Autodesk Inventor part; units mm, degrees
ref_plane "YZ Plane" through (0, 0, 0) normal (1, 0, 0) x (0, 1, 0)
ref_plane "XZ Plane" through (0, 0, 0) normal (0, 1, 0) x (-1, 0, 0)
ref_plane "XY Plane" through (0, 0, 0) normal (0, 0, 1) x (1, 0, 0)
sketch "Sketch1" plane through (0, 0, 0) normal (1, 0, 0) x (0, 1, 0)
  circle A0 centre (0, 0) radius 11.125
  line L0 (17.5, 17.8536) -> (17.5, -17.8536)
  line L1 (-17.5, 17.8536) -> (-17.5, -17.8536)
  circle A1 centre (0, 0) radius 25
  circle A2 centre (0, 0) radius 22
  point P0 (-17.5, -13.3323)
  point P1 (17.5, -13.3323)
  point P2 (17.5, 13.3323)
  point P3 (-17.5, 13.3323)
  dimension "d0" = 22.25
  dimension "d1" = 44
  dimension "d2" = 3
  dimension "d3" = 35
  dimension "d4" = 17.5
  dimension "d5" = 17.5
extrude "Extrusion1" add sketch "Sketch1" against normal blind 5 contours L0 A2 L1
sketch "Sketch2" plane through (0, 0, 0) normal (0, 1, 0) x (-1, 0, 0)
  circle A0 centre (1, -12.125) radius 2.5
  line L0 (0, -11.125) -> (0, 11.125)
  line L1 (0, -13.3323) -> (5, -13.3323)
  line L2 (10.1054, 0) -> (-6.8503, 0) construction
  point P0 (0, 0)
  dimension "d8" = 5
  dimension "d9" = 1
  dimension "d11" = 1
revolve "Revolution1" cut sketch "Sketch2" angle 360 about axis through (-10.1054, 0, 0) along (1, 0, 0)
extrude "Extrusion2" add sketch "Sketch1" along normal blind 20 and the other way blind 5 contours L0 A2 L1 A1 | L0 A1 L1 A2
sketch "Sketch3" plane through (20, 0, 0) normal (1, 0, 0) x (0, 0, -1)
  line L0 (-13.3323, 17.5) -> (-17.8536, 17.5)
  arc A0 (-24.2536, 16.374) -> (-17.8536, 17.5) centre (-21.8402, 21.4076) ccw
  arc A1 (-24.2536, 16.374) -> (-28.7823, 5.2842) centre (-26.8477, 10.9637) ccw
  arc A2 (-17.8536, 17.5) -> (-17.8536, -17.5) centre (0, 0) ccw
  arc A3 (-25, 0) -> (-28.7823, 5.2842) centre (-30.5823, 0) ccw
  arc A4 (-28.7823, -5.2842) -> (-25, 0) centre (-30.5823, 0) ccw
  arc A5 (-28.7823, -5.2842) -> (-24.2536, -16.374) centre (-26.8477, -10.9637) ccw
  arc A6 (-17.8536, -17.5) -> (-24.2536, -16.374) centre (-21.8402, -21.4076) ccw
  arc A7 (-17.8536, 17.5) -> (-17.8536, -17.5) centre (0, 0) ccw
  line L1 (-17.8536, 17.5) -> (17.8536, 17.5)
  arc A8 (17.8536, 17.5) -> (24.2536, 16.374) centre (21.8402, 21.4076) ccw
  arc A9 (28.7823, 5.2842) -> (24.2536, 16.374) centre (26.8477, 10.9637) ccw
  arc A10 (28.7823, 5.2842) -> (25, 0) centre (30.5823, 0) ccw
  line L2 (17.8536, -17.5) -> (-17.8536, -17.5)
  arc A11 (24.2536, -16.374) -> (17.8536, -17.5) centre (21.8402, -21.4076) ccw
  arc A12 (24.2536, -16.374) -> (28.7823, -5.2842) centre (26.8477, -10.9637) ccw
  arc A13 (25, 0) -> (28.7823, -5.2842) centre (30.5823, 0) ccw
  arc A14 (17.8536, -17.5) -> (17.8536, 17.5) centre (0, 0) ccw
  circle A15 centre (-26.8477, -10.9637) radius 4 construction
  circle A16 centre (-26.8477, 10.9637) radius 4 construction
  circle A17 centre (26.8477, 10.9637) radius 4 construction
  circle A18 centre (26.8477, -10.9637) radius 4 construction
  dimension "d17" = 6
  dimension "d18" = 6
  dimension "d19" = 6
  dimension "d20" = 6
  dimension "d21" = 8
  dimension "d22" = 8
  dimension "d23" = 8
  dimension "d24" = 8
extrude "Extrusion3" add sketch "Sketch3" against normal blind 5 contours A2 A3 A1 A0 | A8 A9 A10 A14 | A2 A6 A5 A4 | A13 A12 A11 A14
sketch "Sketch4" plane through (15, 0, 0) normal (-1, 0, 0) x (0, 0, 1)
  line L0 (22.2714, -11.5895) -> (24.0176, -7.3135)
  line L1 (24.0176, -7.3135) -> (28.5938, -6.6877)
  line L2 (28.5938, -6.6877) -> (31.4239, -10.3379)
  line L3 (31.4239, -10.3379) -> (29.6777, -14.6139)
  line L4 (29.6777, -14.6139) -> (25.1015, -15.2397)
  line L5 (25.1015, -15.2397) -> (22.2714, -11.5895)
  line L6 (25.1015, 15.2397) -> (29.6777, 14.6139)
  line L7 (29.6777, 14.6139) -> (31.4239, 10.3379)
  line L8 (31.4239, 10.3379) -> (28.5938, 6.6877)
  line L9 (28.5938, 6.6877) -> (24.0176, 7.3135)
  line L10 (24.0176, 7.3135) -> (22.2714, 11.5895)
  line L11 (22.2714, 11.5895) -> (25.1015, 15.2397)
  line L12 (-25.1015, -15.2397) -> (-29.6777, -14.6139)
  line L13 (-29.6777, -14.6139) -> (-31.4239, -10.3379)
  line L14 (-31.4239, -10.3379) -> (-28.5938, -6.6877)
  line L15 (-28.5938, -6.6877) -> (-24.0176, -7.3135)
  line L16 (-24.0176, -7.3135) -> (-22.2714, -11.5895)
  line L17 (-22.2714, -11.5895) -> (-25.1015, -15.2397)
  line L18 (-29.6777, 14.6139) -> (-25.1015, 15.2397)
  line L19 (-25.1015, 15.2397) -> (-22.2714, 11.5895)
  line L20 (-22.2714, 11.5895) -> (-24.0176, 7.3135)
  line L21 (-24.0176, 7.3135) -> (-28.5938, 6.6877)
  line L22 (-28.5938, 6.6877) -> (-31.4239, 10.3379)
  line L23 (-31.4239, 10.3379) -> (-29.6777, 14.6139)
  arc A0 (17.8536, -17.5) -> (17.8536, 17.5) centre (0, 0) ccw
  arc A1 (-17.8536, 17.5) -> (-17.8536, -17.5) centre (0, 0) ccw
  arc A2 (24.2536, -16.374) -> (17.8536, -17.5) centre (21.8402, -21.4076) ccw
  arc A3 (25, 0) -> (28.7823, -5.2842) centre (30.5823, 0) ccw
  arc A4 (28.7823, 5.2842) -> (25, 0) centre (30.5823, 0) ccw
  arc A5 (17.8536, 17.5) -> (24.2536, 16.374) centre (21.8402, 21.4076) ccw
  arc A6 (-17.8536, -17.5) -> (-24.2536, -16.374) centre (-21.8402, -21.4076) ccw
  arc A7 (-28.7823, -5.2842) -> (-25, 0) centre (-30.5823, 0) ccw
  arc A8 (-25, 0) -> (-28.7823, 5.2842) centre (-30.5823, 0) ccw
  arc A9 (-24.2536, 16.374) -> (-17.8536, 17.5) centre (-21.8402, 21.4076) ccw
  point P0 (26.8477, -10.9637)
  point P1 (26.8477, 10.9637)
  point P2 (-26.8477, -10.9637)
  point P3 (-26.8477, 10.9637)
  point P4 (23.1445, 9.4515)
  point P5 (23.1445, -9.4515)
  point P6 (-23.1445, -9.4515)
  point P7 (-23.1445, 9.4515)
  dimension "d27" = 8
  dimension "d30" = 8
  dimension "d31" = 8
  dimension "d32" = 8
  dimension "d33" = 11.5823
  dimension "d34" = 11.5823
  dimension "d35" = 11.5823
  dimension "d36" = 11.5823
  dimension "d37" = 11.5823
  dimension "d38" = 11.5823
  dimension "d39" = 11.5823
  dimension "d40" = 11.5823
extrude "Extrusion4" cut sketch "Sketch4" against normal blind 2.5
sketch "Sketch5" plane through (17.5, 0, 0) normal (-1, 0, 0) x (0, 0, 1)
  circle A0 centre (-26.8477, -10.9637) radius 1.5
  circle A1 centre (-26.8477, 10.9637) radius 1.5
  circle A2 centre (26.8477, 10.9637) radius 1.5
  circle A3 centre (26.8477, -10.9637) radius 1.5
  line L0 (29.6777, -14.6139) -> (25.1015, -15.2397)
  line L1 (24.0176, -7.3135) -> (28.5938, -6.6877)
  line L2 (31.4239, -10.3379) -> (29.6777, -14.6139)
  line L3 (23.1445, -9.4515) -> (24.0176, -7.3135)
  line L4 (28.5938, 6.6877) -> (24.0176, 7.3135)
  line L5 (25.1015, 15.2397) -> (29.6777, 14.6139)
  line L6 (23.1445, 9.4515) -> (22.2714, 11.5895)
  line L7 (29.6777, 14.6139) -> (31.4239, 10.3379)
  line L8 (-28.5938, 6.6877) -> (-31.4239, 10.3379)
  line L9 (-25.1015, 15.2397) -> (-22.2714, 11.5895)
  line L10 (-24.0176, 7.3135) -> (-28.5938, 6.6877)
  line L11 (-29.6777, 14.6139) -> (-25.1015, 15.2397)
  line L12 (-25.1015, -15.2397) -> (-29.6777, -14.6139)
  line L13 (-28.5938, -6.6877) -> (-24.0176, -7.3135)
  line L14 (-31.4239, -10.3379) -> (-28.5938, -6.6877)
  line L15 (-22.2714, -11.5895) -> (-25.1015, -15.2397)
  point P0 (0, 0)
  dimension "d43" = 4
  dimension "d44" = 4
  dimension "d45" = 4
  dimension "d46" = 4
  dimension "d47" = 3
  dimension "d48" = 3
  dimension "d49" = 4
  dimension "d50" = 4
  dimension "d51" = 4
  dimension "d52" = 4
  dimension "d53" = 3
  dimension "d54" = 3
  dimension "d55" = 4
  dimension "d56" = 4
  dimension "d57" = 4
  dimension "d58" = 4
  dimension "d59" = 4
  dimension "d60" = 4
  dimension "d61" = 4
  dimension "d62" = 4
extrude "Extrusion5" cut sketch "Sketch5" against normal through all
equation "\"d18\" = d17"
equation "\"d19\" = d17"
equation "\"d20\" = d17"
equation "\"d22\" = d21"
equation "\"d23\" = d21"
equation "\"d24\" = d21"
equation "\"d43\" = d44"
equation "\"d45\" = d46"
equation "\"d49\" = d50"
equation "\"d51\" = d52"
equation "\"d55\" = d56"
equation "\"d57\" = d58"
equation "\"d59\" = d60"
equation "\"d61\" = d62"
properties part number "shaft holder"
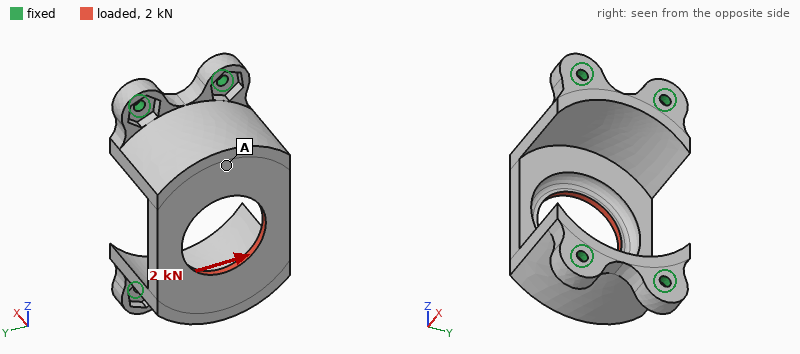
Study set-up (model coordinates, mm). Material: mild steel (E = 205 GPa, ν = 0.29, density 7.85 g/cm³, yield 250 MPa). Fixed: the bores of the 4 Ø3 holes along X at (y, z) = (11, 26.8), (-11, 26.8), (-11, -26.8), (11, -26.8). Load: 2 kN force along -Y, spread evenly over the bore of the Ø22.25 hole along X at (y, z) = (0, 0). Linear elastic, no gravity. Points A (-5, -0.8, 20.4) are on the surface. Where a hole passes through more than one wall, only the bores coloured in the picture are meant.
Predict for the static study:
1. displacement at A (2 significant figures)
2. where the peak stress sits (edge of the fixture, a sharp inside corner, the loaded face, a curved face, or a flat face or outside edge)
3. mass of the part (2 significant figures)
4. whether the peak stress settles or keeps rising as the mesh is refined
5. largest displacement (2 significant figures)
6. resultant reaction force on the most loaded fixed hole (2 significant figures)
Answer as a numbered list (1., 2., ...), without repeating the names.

1. 20 µm
2. edge of the fixture
3. 91 g
4. keeps rising
5. 27 µm
6. 1.2 kN
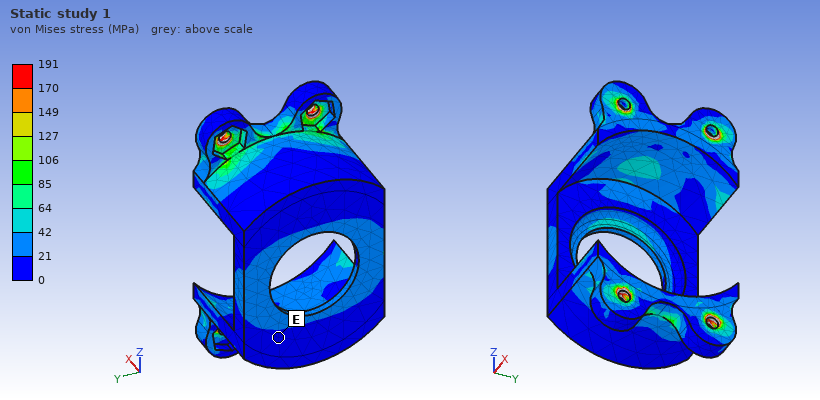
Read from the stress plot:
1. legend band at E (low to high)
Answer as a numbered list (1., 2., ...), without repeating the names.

1. 0 to 21 MPa
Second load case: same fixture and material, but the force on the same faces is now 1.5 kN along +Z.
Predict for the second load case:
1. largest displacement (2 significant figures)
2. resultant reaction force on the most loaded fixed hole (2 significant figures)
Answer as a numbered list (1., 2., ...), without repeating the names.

1. 41 µm
2. 470 N
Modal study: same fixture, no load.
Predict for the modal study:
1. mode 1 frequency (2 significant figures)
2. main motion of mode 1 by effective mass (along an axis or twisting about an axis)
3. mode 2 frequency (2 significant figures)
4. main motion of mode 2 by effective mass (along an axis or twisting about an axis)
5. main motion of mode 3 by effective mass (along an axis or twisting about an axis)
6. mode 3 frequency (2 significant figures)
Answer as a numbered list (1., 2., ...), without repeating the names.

1. 4400 Hz
2. along Z
3. 6700 Hz
4. along Y
5. twisting about X
6. 7600 Hz
